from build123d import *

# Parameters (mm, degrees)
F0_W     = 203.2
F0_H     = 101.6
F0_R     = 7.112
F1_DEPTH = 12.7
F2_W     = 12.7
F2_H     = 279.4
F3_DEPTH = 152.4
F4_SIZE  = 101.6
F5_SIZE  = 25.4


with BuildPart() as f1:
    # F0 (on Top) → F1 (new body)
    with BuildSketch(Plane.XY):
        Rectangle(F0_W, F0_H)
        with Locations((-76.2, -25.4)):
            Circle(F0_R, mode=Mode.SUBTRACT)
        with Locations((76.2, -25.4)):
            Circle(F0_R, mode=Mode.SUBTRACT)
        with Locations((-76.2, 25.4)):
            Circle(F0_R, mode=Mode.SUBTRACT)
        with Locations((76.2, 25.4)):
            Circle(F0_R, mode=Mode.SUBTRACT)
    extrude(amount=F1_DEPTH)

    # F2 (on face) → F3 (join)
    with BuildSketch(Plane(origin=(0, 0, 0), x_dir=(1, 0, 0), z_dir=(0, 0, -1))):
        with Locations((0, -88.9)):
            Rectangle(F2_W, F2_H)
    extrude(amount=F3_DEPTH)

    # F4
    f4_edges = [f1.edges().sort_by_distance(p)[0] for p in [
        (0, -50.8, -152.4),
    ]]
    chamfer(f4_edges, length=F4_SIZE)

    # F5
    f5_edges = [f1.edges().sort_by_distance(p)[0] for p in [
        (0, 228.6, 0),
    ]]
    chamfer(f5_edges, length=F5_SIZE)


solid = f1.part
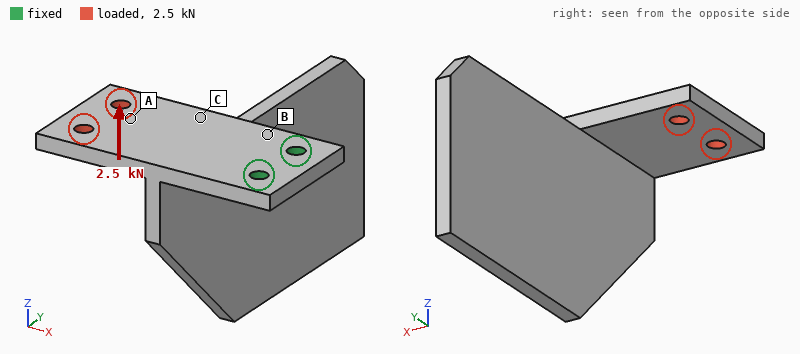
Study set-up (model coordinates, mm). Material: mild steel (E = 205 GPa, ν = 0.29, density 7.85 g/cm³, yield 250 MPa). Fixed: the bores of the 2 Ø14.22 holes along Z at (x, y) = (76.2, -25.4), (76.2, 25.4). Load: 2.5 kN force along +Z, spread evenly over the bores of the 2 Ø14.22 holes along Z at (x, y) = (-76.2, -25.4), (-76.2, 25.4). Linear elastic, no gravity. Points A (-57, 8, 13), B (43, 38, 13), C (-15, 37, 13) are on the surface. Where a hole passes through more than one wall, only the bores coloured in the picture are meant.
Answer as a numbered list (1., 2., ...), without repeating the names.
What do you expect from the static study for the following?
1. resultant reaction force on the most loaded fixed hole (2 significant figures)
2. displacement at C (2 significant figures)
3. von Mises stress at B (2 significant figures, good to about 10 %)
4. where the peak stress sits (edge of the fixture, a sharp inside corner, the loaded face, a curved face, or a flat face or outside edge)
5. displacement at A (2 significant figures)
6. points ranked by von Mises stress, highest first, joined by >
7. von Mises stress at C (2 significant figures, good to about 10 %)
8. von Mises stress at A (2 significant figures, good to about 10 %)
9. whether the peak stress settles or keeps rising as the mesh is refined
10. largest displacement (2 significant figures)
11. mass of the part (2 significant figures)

1. 1.3 kN
2. 0.32 mm
3. 100 MPa
4. edge of the fixture
5. 0.61 mm
6. B > C > A
7. 50 MPa
8. 17 MPa
9. keeps rising
10. 0.94 mm
11. 5.7 kg
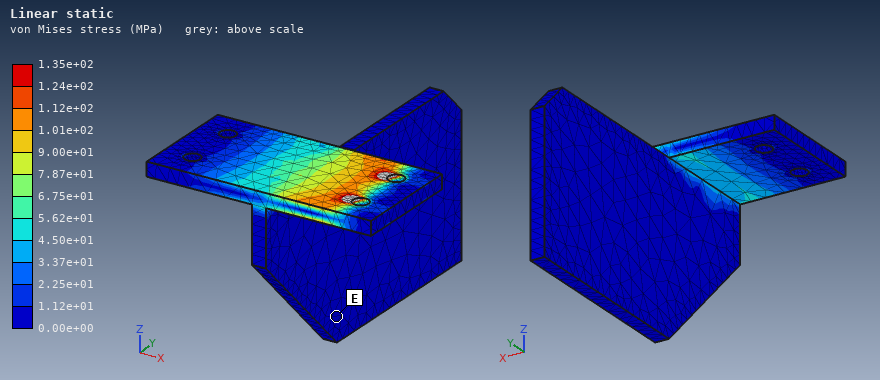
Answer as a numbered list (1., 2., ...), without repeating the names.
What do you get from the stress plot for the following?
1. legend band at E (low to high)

1. 0.00e+00 to 1.12e+01 MPa
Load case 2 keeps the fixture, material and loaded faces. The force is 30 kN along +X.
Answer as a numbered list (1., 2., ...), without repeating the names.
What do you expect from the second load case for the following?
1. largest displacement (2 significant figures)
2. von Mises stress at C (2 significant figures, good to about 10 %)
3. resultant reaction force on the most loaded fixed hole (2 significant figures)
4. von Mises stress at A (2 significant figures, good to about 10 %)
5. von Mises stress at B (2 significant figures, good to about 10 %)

1. 22 µm
2. 24 MPa
3. 15 kN
4. 24 MPa
5. 23 MPa
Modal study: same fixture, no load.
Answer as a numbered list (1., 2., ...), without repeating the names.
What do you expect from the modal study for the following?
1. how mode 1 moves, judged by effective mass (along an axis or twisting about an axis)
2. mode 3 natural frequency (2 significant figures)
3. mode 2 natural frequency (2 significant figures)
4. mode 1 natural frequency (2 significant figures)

1. along X
2. 290 Hz
3. 200 Hz
4. 130 Hz
